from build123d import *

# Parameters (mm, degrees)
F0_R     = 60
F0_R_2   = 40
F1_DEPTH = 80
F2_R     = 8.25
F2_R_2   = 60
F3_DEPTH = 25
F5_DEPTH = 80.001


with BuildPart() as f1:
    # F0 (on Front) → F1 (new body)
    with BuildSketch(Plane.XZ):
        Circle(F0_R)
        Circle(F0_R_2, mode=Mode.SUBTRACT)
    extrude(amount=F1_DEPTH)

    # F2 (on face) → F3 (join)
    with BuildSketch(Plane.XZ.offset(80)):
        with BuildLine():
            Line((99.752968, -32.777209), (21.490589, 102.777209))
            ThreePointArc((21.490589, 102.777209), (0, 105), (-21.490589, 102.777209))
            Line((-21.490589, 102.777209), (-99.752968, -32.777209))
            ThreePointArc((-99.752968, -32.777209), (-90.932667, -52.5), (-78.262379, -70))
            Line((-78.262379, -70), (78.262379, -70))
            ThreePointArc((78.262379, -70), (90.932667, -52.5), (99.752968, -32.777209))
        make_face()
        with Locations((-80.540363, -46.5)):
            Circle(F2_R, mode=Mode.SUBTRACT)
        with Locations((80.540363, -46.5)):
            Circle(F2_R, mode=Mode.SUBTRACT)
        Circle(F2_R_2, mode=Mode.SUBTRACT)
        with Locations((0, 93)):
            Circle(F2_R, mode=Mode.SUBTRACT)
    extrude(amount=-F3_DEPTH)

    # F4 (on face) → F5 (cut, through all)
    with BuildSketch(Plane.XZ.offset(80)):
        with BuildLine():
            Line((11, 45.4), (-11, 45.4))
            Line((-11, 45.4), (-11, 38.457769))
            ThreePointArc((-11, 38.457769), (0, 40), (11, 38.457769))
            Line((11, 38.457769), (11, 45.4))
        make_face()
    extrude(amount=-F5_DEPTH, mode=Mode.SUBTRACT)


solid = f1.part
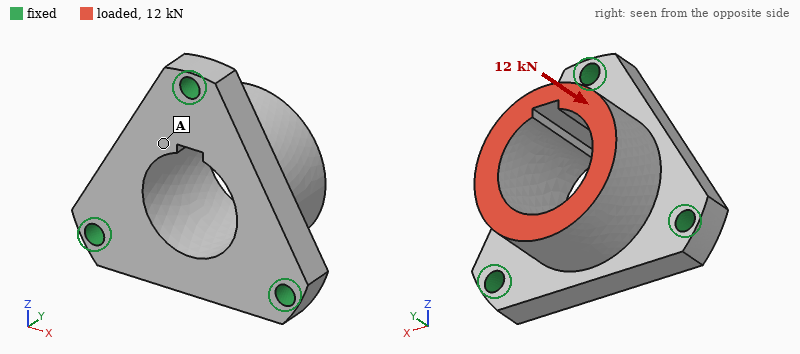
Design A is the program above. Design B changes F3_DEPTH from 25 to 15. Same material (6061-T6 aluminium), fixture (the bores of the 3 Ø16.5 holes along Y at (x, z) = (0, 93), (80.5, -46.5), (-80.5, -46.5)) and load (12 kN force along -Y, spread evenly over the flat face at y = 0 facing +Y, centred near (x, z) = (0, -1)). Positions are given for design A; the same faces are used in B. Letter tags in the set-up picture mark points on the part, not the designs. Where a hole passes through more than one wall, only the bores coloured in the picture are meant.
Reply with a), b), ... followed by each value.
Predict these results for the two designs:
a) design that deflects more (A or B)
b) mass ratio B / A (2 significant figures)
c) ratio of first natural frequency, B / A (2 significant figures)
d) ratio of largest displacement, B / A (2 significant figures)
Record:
a) B
b) 0.85
c) 0.69
d) 2.2
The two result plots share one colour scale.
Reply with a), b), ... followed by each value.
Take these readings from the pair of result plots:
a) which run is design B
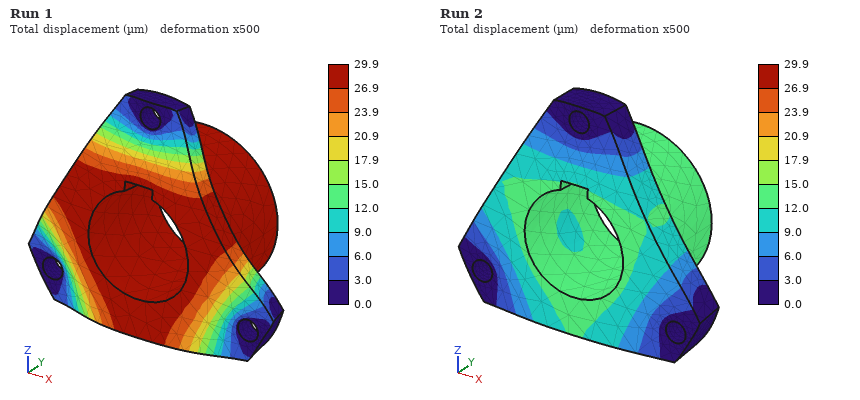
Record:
a) Run 1
